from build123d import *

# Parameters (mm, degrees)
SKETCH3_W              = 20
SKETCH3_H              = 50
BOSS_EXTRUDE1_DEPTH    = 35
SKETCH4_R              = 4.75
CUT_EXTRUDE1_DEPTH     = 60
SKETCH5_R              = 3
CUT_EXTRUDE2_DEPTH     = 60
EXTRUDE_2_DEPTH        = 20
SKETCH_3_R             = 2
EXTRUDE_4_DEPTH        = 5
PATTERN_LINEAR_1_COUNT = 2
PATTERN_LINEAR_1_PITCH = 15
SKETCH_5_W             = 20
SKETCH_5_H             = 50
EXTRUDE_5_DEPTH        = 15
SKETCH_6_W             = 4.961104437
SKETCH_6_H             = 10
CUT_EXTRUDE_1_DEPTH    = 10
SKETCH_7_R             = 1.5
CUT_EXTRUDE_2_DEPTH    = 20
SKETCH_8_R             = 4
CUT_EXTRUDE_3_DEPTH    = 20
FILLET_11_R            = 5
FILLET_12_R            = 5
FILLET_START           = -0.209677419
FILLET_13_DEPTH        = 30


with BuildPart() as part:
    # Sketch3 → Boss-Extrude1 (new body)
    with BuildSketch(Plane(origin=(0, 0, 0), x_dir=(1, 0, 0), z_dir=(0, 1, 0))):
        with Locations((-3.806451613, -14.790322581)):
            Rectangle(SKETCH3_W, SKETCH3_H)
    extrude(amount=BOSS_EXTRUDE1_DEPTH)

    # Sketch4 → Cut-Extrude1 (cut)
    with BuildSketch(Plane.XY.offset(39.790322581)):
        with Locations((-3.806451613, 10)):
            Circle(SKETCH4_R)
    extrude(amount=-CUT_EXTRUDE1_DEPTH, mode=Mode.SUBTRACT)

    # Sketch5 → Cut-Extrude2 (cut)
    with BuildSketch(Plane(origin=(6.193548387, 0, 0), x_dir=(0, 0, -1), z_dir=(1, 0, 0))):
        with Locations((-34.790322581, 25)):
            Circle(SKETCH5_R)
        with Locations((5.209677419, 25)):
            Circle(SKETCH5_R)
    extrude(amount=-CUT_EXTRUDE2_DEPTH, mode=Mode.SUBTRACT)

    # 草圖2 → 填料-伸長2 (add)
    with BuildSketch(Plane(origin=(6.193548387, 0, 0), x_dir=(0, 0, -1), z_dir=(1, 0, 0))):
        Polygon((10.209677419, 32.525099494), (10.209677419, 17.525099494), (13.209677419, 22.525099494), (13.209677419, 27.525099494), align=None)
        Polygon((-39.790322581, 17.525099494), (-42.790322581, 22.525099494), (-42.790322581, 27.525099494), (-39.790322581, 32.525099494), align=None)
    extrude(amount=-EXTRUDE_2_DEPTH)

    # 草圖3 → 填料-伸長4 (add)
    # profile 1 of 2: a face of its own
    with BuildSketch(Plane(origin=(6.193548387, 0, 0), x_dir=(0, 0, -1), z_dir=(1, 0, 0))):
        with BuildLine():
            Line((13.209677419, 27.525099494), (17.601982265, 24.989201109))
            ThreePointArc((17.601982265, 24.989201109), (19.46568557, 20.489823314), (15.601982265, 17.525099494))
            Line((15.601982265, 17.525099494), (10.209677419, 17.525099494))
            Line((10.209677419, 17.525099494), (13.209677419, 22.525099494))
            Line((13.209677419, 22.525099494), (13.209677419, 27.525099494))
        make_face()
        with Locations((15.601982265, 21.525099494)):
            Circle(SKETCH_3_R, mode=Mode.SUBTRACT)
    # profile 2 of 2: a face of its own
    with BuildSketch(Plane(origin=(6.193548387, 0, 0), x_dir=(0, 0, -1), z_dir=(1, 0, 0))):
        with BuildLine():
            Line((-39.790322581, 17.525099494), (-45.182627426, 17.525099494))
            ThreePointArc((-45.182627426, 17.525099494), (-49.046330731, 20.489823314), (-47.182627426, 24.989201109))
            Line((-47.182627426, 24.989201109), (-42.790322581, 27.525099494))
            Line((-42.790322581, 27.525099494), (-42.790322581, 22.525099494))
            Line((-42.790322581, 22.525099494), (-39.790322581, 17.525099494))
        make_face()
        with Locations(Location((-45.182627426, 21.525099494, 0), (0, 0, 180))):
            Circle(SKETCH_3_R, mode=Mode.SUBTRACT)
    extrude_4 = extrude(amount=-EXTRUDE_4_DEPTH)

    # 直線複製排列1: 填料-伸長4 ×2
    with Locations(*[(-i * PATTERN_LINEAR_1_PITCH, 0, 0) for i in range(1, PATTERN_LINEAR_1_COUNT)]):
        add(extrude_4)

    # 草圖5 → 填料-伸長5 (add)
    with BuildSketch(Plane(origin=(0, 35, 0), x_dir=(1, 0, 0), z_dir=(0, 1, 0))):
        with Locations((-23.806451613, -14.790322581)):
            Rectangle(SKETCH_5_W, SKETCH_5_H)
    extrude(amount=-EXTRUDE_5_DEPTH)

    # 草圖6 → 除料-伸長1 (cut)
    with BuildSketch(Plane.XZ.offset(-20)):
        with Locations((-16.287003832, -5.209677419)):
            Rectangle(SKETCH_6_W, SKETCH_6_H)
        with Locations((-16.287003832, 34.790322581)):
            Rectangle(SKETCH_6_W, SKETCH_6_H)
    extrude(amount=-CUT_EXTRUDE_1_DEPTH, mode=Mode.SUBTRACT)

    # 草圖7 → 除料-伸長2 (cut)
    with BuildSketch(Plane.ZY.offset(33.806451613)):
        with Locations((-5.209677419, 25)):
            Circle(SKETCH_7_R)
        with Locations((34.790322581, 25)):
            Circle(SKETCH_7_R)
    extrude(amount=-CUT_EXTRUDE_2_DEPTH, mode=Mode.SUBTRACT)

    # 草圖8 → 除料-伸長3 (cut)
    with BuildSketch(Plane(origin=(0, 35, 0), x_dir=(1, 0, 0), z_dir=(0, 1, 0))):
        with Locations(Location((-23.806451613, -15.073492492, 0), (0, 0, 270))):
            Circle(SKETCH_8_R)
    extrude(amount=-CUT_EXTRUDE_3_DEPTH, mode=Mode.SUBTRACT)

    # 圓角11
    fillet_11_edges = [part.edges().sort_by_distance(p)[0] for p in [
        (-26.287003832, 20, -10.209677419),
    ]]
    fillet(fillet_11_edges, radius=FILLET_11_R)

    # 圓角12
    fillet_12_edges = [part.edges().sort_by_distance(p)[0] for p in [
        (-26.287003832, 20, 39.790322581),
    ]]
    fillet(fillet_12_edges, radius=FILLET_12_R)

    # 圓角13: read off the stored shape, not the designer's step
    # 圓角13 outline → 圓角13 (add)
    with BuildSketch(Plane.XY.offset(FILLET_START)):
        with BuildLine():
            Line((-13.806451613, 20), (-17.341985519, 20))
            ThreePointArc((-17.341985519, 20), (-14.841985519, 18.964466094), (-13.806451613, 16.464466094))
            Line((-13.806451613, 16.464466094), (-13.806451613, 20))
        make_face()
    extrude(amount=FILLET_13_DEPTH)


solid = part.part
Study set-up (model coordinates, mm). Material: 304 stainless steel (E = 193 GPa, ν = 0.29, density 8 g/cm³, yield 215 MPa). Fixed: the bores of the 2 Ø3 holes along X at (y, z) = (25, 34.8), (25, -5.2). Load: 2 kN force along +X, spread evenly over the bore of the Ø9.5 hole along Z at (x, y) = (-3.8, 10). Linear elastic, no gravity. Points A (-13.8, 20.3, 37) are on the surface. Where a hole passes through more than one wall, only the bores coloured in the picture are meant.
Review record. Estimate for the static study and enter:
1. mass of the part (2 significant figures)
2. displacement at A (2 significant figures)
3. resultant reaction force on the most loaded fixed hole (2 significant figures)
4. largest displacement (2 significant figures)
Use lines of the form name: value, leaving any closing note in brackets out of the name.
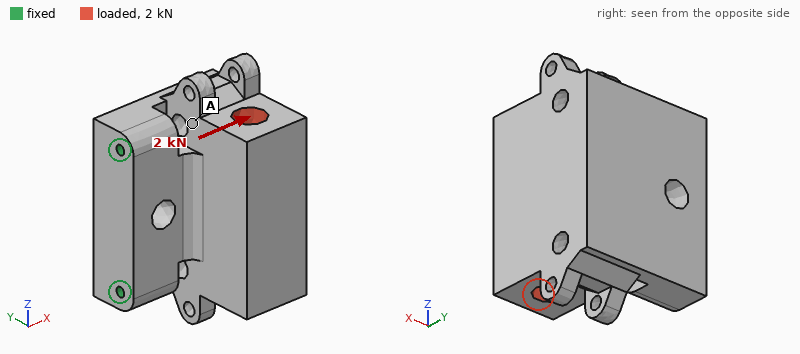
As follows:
mass of the part: 360 g
displacement at A: 6.3 µm
resultant reaction force on the most loaded fixed hole: 1.0 kN
largest displacement: 23 µm
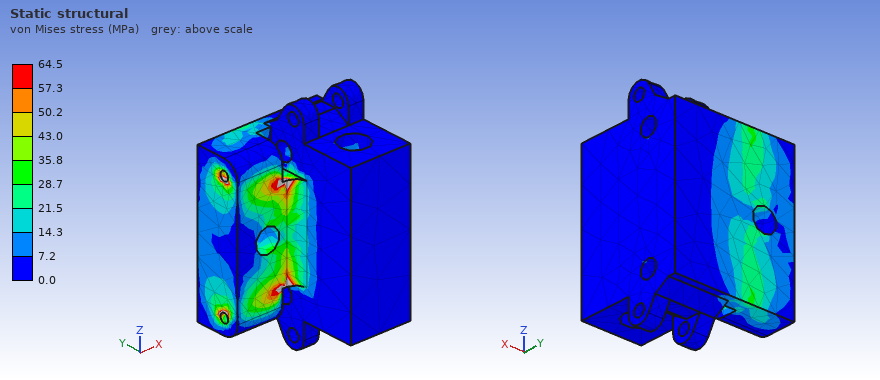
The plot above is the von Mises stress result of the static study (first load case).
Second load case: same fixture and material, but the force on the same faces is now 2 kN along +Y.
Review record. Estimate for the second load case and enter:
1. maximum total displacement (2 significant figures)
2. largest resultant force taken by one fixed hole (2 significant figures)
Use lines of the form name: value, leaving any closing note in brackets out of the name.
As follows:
maximum total displacement: 23 µm
largest resultant force taken by one fixed hole: 1.1 kN
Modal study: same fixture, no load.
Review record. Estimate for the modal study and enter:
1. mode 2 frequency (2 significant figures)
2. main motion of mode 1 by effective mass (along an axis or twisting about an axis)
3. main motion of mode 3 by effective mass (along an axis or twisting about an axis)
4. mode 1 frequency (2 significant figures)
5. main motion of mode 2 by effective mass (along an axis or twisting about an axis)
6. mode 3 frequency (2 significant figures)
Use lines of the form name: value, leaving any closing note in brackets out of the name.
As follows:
mode 2 frequency: 6400 Hz
main motion of mode 1 by effective mass: along Y
main motion of mode 3 by effective mass: along Z
mode 1 frequency: 3300 Hz
main motion of mode 2 by effective mass: along Z
mode 3 frequency: 9400 Hz
